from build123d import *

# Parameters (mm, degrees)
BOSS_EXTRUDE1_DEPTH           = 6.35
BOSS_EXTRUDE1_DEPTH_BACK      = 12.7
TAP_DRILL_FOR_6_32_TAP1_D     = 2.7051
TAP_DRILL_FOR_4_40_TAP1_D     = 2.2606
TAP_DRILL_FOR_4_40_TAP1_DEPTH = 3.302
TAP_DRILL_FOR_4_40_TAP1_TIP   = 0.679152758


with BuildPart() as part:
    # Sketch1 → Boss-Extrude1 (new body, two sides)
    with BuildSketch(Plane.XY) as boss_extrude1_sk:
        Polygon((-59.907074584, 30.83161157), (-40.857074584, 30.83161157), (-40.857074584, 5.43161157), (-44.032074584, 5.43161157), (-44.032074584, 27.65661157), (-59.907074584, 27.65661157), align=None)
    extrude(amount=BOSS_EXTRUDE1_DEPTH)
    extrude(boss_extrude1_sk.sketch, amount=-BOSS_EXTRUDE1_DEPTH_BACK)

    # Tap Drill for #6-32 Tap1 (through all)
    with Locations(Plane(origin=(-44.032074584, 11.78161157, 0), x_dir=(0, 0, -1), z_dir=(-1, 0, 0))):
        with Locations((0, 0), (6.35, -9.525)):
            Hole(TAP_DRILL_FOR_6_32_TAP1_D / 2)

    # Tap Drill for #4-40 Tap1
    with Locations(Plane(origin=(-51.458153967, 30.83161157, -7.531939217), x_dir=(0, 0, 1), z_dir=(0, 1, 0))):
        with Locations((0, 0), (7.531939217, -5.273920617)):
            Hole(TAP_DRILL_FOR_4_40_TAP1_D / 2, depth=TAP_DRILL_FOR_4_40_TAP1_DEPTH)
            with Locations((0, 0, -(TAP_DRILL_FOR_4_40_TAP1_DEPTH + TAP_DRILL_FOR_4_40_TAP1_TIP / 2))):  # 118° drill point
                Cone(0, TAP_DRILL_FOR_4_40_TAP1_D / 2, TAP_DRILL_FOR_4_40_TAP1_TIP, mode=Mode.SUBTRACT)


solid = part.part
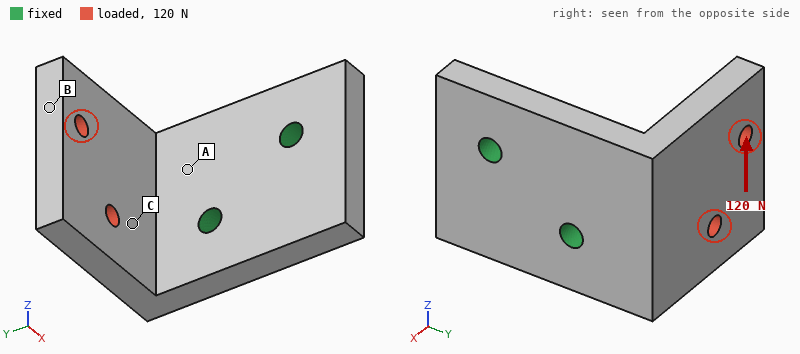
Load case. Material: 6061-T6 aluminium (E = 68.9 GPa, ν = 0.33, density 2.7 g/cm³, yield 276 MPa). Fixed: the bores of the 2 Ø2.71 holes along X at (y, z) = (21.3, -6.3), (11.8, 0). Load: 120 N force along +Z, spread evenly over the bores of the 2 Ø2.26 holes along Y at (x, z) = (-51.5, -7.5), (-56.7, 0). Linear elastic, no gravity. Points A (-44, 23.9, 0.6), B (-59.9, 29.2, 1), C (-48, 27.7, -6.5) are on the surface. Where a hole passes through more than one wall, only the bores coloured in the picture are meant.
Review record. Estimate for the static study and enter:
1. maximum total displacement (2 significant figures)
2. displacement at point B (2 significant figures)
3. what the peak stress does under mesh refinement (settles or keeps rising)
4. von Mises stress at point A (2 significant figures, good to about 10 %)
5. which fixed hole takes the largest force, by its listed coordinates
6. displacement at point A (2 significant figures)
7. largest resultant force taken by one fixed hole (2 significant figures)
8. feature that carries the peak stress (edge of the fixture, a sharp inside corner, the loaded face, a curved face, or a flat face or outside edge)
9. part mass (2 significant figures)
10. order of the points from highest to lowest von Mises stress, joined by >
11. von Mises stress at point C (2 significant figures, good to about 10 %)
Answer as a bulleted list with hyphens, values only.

- 45 µm
- 39 µm
- keeps rising
- 21 MPa
- (21.3, -6.3)
- 8.2 µm
- 170 N
- edge of the fixture
- 6.6 g
- A > C > B
- 13 MPa
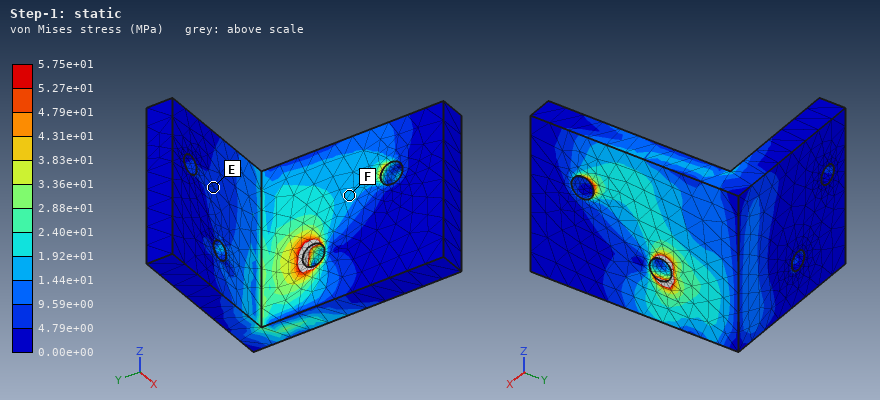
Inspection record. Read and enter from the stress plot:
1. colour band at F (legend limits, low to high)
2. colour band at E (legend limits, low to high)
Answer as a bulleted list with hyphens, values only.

- 1.44e+01 to 1.92e+01 MPa
- 4.79e+00 to 9.59e+00 MPa
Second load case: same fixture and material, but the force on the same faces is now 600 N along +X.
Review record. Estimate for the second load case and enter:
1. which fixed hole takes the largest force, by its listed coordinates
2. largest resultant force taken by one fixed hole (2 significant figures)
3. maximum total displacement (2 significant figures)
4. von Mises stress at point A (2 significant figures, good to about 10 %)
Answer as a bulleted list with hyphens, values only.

- (21.3, -6.3)
- 690 N
- 0.14 mm
- 63 MPa
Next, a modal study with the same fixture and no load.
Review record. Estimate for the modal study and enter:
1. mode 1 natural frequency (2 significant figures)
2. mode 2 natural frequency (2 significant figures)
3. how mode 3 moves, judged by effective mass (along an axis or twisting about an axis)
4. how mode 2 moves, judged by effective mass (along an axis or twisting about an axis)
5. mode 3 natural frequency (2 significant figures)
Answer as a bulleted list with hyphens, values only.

- 4800 Hz
- 6700 Hz
- along X
- along Z
- 15 kHz
